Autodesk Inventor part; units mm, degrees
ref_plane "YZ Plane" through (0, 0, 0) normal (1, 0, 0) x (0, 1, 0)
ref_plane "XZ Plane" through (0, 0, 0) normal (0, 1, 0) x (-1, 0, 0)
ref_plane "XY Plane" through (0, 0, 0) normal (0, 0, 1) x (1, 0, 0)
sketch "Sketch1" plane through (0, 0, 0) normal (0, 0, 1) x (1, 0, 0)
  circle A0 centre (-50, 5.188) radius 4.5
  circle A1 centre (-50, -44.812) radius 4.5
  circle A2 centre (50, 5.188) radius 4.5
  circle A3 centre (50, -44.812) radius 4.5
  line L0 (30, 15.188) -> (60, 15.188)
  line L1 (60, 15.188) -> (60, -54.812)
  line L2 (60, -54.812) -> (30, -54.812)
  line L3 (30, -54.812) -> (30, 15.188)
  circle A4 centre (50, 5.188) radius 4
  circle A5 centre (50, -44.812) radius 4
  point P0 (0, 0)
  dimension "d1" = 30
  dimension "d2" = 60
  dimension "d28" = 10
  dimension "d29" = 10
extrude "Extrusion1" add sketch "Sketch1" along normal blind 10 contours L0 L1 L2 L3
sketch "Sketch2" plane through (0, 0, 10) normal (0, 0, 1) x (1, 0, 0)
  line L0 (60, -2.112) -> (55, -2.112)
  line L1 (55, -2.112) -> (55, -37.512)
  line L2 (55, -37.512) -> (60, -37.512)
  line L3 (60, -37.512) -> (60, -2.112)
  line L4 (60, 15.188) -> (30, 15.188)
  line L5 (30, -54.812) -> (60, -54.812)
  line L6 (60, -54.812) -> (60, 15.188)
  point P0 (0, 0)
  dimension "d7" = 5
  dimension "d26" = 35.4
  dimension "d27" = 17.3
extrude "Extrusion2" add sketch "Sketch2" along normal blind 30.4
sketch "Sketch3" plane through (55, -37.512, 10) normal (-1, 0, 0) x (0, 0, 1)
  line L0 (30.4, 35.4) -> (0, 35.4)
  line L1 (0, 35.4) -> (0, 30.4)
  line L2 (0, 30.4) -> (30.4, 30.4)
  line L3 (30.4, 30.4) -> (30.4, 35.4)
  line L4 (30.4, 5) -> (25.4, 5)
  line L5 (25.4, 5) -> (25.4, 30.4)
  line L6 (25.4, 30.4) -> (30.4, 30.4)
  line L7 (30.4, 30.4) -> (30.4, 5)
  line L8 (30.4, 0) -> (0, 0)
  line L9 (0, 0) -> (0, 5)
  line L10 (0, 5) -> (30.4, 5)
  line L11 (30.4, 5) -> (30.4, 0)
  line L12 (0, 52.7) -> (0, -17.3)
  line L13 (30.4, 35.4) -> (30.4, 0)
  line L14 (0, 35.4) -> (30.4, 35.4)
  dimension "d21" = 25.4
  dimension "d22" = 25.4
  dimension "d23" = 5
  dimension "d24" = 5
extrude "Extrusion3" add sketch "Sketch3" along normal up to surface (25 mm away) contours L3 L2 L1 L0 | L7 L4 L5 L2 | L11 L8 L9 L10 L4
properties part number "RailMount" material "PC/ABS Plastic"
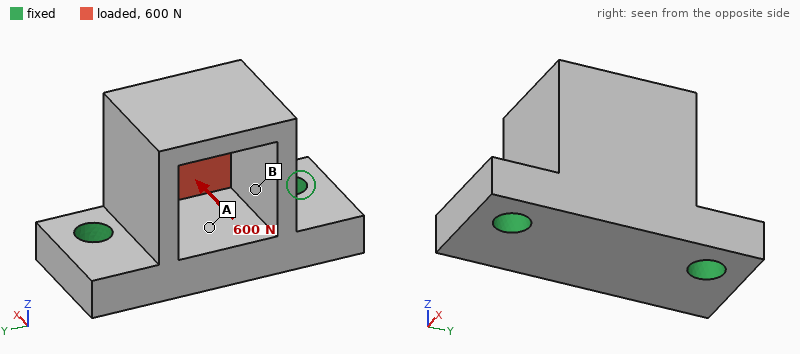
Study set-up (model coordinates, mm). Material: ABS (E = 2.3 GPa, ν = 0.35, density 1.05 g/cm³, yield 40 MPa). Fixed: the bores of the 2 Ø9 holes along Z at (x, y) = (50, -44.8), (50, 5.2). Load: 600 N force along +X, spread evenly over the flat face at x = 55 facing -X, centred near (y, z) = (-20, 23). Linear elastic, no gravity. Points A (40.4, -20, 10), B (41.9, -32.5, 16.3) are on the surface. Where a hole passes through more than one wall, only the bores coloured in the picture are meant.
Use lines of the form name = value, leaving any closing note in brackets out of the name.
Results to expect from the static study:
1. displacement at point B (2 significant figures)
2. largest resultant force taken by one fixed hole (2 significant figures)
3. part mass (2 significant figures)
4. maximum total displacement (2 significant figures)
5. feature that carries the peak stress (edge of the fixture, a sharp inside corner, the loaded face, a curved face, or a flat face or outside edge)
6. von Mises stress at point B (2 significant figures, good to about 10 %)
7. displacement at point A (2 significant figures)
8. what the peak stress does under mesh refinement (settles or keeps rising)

displacement at point B = 0.10 mm
largest resultant force taken by one fixed hole = 310 N
part mass = 38 g
maximum total displacement = 0.32 mm
feature that carries the peak stress = edge of the fixture
von Mises stress at point B = 2.3 MPa
displacement at point A = 0.079 mm
what the peak stress does under mesh refinement = keeps rising
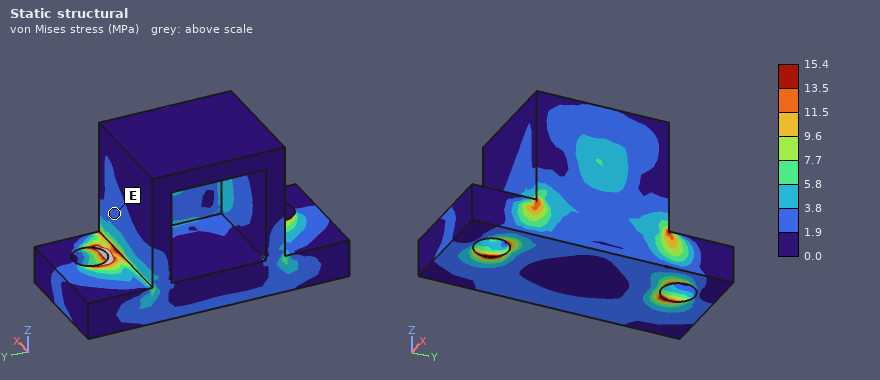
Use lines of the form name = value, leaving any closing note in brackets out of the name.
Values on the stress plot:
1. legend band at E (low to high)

legend band at E = 1.9 to 3.8 MPa
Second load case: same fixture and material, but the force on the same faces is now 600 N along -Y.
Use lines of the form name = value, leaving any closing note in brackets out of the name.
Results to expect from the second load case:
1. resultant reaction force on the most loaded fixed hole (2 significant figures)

resultant reaction force on the most loaded fixed hole = 400 N
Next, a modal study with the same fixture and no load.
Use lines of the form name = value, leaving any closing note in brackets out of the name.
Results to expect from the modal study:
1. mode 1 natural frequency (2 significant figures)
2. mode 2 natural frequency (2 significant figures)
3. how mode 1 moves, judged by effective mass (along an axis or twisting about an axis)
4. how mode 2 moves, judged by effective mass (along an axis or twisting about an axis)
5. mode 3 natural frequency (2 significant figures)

mode 1 natural frequency = 1600 Hz
mode 2 natural frequency = 1900 Hz
how mode 1 moves, judged by effective mass = along X
how mode 2 moves, judged by effective mass = along Y
mode 3 natural frequency = 4100 Hz
